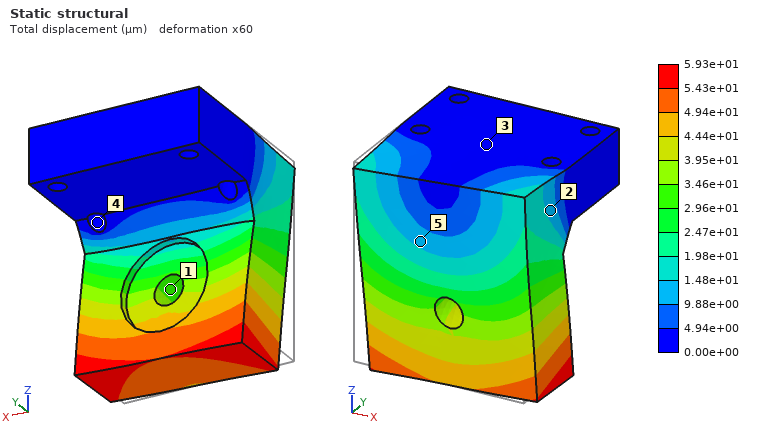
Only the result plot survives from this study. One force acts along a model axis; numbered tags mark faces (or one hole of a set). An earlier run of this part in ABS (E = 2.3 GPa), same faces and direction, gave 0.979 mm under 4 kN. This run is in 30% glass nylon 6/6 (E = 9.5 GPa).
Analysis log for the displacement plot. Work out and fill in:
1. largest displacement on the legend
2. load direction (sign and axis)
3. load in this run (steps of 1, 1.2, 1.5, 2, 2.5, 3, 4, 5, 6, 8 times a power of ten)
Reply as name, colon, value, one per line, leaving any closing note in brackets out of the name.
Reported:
largest displacement on the legend: 5.93e+01 µm
load direction: +X
load in this run: 1 kN
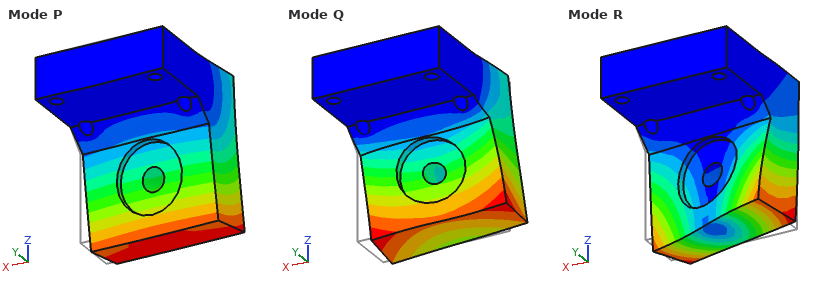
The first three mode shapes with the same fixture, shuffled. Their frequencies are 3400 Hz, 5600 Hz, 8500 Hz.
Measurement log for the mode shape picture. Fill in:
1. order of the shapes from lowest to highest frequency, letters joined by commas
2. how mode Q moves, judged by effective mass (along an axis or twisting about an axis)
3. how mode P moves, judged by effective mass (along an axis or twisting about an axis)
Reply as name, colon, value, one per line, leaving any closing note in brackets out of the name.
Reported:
order of the shapes from lowest to highest frequency, letters joined by commas: P, Q, R
how mode Q moves, judged by effective mass: along X
how mode P moves, judged by effective mass: along Y
